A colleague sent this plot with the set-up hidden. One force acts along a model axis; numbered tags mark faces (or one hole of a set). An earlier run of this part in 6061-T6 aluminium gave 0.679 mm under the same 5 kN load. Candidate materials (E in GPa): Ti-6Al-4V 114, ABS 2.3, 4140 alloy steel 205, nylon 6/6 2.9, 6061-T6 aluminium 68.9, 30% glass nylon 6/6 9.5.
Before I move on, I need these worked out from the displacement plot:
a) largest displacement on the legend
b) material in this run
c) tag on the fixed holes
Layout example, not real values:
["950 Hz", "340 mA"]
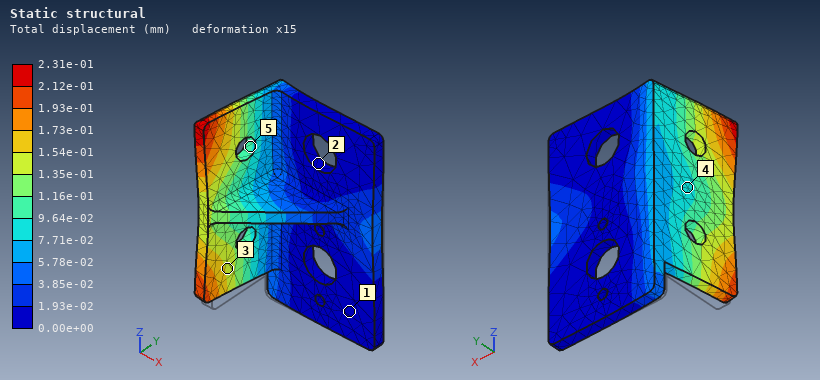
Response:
["2.31e-01 mm", "4140 alloy steel", "2"]
